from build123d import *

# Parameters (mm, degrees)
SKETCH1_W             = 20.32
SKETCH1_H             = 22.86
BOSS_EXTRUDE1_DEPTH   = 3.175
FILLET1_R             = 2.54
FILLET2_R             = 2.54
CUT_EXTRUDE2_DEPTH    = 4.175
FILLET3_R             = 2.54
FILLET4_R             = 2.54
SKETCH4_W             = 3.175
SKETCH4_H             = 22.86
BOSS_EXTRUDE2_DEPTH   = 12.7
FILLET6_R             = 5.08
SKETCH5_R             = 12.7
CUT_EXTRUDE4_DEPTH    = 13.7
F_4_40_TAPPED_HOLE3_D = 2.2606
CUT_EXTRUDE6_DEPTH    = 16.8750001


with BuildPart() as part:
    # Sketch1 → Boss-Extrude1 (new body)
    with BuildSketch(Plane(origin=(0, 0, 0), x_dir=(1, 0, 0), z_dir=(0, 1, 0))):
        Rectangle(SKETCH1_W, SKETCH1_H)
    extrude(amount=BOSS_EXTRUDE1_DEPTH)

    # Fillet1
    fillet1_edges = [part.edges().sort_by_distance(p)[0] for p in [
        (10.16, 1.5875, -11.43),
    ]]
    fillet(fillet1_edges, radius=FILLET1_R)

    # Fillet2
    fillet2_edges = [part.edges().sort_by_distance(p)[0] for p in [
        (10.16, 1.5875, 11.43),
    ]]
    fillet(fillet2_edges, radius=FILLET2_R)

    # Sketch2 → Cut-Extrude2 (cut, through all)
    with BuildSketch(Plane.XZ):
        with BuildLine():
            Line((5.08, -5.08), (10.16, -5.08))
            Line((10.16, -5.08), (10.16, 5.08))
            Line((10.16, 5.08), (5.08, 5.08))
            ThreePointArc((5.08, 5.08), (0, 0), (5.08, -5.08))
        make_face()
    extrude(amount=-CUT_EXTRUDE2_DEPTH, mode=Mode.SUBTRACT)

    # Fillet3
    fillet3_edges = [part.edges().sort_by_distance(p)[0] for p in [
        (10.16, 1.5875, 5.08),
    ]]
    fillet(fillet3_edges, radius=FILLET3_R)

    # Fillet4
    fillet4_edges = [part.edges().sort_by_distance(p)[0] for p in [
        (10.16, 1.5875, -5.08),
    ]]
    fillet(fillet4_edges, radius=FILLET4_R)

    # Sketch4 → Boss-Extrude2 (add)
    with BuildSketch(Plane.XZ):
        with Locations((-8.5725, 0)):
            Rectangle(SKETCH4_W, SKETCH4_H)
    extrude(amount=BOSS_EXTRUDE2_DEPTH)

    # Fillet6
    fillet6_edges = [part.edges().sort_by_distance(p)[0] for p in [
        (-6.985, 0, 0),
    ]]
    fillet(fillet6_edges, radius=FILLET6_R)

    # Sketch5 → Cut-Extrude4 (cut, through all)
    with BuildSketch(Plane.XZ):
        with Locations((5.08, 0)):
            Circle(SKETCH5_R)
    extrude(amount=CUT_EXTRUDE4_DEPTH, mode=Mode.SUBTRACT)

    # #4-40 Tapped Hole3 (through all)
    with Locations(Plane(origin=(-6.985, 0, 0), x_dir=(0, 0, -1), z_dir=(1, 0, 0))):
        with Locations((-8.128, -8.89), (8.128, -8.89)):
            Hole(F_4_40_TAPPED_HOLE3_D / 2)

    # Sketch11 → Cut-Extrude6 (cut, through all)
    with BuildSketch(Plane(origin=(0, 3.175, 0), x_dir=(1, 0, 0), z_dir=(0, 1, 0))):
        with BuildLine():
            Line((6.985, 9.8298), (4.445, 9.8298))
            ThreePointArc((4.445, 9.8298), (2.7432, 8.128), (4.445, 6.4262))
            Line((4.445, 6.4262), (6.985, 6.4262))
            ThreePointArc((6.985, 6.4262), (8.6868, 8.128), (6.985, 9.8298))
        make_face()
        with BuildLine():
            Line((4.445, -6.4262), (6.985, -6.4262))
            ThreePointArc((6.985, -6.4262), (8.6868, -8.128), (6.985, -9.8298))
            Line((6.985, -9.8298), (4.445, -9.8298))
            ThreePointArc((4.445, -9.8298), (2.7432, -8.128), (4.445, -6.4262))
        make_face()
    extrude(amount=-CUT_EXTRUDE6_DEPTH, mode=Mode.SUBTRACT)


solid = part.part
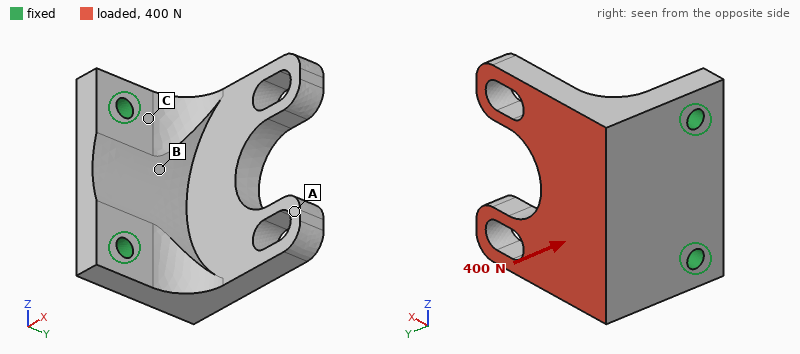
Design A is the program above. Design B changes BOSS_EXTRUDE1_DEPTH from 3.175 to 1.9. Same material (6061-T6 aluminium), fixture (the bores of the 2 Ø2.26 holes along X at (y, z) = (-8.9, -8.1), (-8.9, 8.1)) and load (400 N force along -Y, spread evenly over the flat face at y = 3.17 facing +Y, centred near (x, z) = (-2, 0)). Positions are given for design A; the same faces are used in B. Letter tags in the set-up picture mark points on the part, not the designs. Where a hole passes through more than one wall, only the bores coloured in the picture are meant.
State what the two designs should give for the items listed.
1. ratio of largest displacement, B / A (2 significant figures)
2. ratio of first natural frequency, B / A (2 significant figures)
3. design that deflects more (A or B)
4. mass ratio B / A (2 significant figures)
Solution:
1.7
1.1
B
0.78
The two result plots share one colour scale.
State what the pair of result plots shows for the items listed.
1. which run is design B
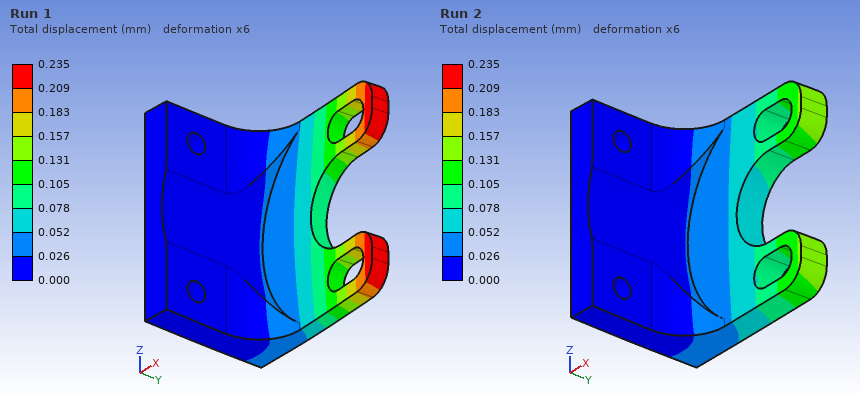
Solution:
Run 1
